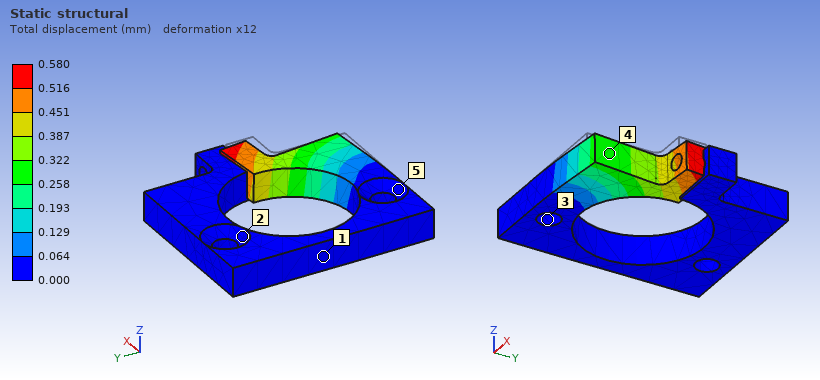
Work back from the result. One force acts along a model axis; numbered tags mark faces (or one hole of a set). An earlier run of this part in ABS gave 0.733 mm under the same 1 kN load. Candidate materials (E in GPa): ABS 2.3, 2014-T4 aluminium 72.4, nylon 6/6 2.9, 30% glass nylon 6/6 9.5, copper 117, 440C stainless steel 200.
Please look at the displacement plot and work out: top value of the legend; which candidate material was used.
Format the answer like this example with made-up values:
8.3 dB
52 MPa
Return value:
0.580 mm
nylon 6/6
